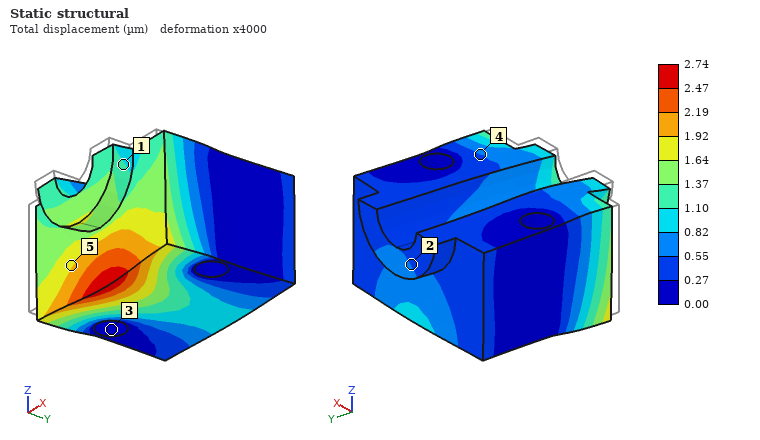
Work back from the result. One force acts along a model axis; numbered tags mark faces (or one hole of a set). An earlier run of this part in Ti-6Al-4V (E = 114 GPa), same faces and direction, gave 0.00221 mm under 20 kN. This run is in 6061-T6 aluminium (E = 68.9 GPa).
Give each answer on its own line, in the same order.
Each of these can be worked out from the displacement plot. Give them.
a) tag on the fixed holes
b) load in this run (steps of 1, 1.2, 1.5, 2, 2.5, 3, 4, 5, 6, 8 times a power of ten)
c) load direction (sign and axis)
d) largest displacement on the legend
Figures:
3
15 kN
+Y
2.74 µm
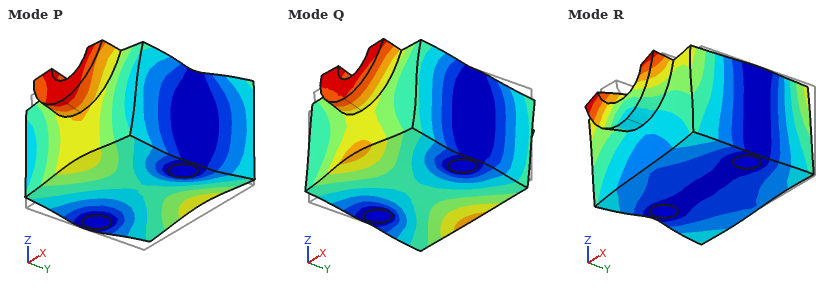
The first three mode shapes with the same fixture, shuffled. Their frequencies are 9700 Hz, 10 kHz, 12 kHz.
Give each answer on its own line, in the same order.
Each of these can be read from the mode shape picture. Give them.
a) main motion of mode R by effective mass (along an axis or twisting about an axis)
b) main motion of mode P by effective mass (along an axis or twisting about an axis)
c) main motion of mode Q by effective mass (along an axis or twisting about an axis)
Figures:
along X
along Z
twisting about X
